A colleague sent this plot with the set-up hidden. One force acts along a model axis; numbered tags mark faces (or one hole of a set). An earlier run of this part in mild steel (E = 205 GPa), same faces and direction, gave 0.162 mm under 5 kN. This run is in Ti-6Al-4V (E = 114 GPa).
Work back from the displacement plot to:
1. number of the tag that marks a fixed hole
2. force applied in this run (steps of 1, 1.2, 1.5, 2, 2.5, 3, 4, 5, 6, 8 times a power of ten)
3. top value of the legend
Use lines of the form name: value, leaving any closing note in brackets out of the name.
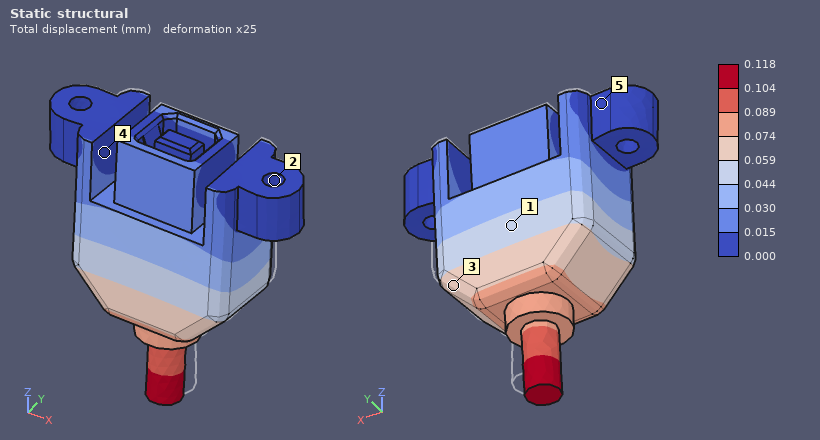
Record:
number of the tag that marks a fixed hole: 2
force applied in this run: 2 kN
top value of the legend: 0.118 mm
